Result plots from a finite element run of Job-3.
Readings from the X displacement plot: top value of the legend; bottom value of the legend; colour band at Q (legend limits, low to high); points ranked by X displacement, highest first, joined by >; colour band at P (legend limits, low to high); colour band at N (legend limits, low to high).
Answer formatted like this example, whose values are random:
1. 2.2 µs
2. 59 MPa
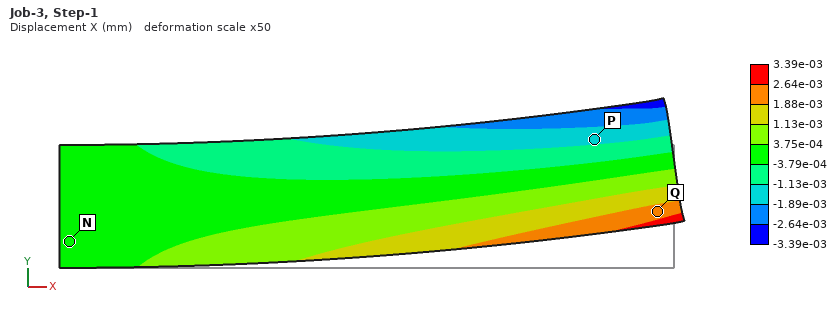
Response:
1. 3.39e-03 mm
2. -3.39e-03 mm
3. 1.88e-03 to 2.64e-03 mm
4. Q > N > P
5. -1.89e-03 to -1.13e-03 mm
6. -3.79e-04 to 3.75e-04 mm
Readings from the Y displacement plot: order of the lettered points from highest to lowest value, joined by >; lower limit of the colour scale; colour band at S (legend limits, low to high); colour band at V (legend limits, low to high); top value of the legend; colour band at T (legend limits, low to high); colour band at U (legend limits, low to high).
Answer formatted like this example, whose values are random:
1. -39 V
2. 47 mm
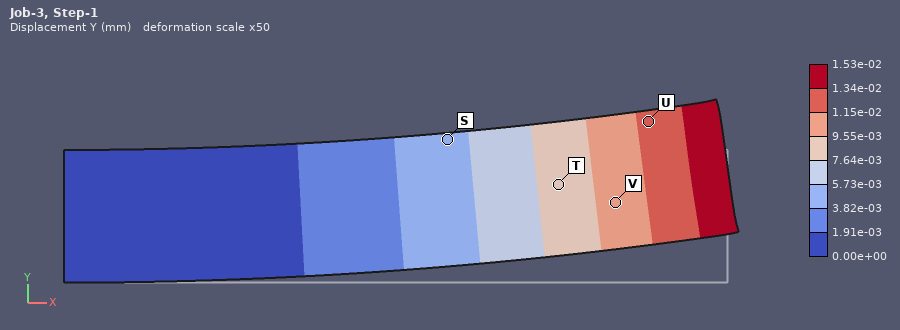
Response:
1. U > V > T > S
2. 0.00e+00 mm
3. 3.82e-03 to 5.73e-03 mm
4. 9.55e-03 to 1.15e-02 mm
5. 1.53e-02 mm
6. 7.64e-03 to 9.55e-03 mm
7. 1.15e-02 to 1.34e-02 mm
